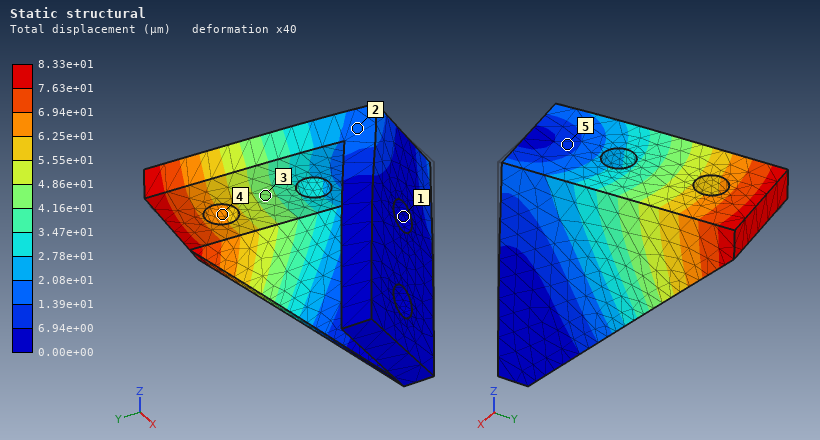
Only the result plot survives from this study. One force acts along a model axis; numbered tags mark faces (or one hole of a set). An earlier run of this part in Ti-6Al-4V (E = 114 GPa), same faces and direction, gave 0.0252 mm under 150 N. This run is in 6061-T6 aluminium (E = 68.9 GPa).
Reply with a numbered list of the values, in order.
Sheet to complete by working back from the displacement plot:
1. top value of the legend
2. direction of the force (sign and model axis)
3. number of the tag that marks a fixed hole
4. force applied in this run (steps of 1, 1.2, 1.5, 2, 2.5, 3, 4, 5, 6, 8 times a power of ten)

1. 8.33e+01 µm
2. -X
3. 1
4. 300 N
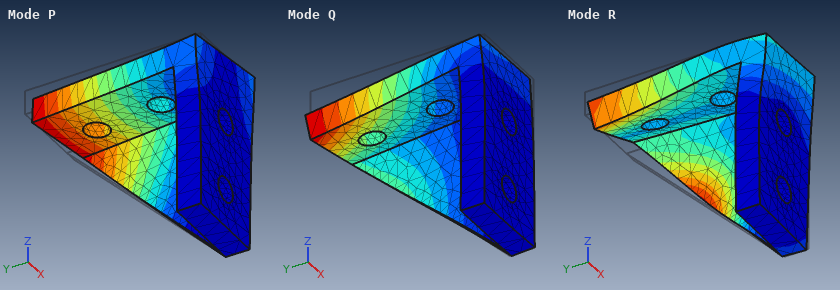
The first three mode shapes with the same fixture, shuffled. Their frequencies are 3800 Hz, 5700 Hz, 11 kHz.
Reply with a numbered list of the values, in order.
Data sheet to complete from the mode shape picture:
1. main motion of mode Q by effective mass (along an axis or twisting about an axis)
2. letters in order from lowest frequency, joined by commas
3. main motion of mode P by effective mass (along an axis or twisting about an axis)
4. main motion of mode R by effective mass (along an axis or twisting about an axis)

1. along Z
2. P, Q, R
3. along X
4. along Y
